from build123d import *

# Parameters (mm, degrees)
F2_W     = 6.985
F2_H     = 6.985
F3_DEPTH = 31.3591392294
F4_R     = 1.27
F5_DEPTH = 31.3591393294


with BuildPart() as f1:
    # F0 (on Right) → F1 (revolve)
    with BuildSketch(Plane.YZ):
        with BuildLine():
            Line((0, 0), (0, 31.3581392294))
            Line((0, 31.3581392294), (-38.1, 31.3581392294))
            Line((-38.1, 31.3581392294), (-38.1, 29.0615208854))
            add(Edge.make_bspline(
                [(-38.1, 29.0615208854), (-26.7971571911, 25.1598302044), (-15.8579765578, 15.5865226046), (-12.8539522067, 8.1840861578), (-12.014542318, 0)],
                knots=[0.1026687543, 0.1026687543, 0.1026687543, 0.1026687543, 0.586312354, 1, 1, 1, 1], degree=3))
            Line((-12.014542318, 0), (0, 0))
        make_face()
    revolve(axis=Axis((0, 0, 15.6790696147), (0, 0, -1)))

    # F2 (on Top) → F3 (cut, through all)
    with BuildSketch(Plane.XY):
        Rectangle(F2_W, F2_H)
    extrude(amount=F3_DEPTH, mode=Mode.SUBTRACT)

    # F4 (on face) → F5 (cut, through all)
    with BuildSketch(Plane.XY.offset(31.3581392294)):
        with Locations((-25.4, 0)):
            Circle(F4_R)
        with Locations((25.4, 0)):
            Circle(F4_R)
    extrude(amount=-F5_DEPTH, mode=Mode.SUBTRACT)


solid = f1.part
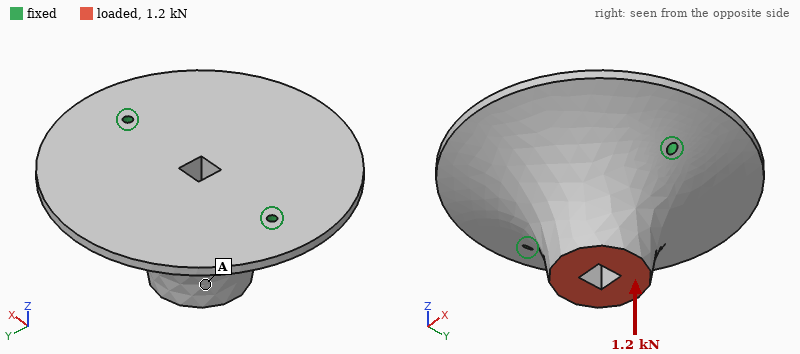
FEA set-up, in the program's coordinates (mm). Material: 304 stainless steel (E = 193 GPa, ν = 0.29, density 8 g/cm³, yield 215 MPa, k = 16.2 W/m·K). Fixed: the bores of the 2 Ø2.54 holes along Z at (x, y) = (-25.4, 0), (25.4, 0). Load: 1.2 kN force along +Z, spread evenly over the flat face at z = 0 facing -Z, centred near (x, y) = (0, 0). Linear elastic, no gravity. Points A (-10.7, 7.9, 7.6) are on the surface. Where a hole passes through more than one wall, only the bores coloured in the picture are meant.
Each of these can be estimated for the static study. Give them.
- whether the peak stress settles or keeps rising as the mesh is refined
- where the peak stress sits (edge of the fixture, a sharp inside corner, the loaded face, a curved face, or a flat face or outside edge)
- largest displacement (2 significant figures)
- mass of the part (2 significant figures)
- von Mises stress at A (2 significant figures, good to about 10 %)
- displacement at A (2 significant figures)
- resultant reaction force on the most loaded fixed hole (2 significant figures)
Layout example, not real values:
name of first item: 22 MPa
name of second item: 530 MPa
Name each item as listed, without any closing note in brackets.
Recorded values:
whether the peak stress settles or keeps rising as the mesh is refined: keeps rising
where the peak stress sits: edge of the fixture
largest displacement: 1.4 µm
mass of the part: 380 g
von Mises stress at A: 3.2 MPa
displacement at A: 1.1 µm
resultant reaction force on the most loaded fixed hole: 690 N
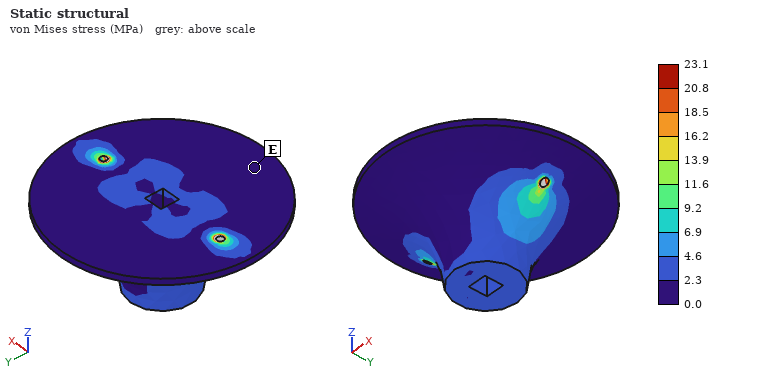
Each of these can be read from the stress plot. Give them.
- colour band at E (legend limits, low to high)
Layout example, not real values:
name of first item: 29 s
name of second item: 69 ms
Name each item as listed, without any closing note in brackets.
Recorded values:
colour band at E: 0.0 to 2.3 MPa
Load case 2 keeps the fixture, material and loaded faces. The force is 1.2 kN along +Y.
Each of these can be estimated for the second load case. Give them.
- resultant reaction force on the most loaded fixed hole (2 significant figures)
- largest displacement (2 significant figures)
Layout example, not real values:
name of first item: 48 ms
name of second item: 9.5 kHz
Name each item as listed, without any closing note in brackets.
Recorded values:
resultant reaction force on the most loaded fixed hole: 600 N
largest displacement: 24 µm
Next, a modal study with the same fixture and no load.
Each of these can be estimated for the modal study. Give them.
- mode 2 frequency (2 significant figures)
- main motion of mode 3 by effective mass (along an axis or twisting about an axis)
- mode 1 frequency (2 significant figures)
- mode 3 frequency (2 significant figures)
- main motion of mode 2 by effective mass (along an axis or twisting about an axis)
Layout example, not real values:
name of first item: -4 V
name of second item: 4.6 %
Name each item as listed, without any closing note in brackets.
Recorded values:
mode 2 frequency: 8800 Hz
main motion of mode 3 by effective mass: twisting about Y
mode 1 frequency: 3500 Hz
mode 3 frequency: 14 kHz
main motion of mode 2 by effective mass: along Z
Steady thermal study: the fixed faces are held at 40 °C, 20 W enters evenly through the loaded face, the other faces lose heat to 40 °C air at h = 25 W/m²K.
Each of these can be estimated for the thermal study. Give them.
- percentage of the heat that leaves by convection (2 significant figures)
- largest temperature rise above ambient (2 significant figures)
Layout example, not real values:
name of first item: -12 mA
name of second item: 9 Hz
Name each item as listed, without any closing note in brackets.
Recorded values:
percentage of the heat that leaves by convection: 35 %
largest temperature rise above ambient: 70 K
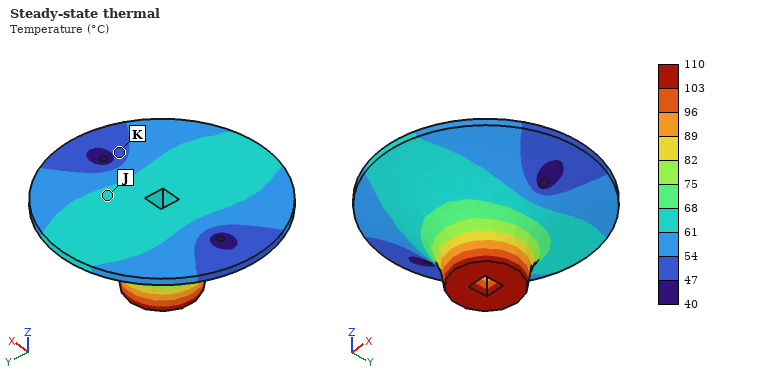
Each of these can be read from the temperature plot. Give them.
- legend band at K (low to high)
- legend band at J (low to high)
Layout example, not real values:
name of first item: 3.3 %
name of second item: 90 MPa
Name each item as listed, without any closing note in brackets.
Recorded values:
legend band at K: 47 to 54 °C
legend band at J: 61 to 68 °C
